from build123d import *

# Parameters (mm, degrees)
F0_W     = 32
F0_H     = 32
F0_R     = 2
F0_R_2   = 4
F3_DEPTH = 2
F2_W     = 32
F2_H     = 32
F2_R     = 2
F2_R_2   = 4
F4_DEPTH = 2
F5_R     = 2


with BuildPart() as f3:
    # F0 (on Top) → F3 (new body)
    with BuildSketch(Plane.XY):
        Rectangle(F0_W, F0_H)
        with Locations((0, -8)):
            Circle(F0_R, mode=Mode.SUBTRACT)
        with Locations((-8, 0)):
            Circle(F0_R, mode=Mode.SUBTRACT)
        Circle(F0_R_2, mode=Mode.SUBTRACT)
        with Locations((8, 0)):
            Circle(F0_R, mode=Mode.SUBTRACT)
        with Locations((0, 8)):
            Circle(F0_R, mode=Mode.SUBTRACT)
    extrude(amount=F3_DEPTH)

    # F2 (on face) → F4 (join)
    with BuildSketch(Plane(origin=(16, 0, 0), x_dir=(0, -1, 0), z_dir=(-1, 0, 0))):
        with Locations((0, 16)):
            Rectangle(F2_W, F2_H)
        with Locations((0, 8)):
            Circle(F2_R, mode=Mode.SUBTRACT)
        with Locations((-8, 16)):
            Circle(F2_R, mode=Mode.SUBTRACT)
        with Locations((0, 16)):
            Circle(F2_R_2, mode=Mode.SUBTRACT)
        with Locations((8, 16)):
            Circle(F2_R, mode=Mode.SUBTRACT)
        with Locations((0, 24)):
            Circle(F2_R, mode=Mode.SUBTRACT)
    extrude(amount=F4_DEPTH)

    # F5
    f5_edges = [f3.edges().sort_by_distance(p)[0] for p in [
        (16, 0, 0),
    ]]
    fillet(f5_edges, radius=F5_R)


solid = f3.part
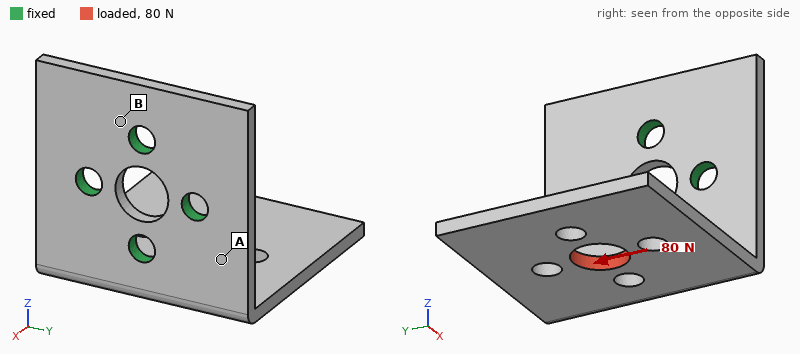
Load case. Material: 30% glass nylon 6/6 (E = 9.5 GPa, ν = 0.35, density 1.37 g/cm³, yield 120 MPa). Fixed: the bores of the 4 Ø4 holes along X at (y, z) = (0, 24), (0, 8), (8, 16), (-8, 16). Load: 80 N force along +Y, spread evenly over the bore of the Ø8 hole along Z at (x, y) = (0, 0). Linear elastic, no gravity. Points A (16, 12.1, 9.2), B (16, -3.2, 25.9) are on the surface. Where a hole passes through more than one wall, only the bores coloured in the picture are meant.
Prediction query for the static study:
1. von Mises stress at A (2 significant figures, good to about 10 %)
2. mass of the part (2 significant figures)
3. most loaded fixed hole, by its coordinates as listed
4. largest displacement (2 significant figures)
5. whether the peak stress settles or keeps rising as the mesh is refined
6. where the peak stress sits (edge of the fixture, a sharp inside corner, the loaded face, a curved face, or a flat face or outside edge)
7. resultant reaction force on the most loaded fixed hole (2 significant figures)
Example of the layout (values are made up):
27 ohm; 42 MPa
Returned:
18 MPa; 4.8 g; (0, 8); 0.65 mm; keeps rising; edge of the fixture; 72 N
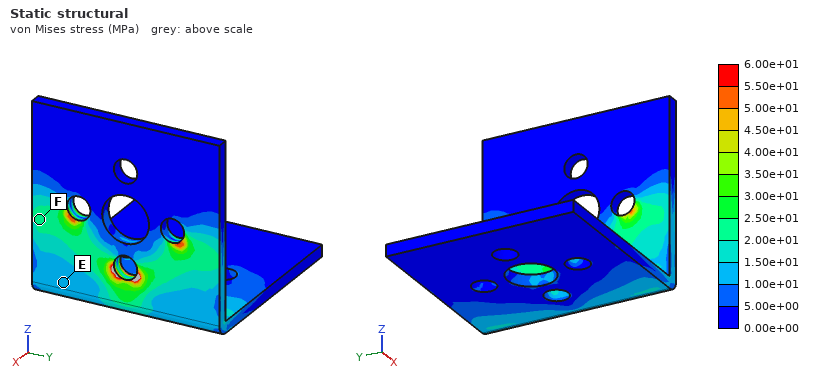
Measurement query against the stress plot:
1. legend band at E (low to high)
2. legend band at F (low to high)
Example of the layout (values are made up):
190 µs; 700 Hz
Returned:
1.00e+01 to 1.50e+01 MPa; 2.00e+01 to 2.50e+01 MPa
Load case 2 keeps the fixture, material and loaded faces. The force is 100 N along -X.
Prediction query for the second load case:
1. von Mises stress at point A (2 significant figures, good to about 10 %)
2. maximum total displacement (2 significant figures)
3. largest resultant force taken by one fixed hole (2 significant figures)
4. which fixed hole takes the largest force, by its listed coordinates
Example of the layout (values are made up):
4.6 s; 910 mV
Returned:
7.4 MPa; 0.38 mm; 110 N; (0, 8)
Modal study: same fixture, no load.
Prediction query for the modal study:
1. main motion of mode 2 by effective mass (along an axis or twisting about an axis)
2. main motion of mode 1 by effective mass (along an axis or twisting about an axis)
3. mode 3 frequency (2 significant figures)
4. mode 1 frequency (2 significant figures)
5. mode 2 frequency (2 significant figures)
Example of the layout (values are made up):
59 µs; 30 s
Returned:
along Y; along Z; 1900 Hz; 670 Hz; 1200 Hz
